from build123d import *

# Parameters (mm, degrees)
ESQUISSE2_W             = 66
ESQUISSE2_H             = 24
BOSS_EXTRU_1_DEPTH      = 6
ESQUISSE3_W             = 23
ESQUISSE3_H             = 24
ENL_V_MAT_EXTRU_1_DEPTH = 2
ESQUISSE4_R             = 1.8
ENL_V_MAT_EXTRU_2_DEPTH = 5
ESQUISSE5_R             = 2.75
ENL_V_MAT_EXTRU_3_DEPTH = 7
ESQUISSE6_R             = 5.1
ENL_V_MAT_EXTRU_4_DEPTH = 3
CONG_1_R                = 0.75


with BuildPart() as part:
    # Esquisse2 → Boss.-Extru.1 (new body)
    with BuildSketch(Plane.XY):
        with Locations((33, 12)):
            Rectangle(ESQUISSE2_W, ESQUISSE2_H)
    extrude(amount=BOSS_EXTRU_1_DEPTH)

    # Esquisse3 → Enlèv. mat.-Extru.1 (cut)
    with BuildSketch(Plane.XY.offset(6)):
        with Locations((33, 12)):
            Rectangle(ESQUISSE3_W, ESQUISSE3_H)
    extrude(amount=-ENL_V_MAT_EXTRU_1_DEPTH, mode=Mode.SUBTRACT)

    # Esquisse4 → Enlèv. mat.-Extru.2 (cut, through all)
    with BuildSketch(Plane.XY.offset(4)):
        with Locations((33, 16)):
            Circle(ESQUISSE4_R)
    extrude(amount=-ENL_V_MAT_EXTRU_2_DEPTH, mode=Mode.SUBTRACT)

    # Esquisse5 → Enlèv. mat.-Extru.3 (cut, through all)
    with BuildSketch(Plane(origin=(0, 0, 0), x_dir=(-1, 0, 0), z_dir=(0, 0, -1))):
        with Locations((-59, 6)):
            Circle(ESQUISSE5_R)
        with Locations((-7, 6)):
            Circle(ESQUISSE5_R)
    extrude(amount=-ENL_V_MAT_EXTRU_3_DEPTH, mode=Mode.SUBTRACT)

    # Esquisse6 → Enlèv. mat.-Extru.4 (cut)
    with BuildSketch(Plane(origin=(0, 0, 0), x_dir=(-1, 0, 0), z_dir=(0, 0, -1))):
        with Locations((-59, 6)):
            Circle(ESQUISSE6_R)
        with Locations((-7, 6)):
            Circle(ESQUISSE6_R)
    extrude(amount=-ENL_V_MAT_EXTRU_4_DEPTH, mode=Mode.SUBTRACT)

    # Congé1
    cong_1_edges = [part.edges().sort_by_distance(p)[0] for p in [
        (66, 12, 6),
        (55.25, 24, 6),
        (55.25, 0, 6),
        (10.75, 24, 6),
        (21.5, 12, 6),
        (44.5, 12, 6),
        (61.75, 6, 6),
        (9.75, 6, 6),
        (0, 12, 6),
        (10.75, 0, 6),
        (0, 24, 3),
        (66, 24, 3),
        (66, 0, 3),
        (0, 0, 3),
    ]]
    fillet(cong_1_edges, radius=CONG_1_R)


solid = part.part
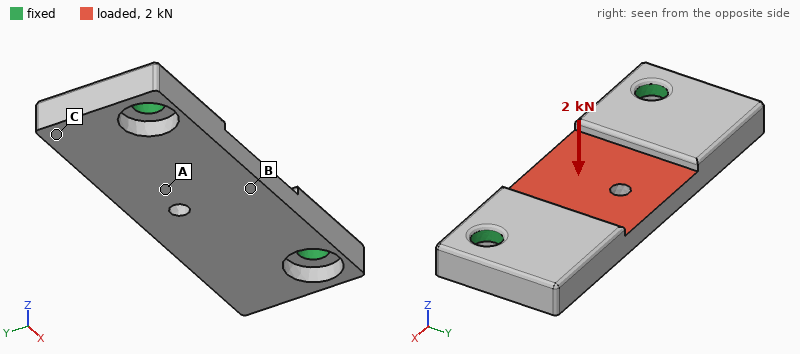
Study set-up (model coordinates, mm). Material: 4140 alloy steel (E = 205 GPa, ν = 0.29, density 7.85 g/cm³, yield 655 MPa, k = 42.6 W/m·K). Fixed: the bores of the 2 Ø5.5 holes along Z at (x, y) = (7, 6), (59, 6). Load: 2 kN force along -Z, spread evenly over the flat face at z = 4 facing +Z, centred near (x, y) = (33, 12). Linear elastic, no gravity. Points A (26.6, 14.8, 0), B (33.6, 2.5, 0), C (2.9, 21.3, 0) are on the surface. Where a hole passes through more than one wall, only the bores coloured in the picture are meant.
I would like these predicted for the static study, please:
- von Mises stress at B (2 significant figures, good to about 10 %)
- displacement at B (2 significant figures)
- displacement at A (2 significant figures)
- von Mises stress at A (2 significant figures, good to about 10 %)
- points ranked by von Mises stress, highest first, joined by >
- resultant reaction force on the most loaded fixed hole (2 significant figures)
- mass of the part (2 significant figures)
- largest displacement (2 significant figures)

140 MPa
36 µm
50 µm
80 MPa
B > A > C
2.3 kN
60 g
72 µm
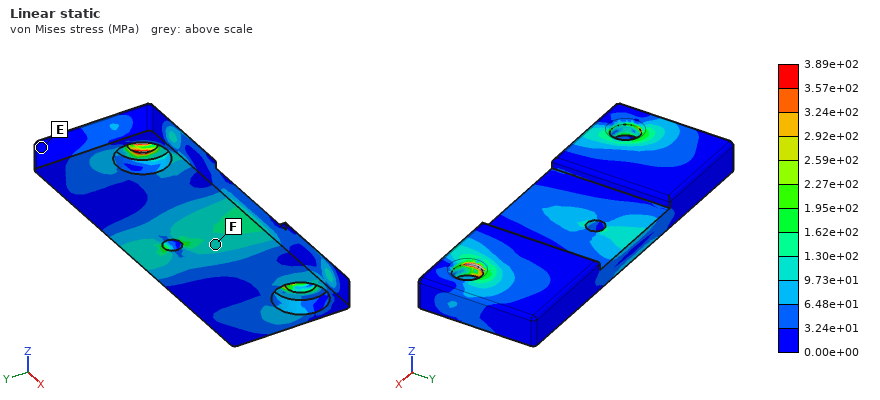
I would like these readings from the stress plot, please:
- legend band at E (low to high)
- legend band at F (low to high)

0.00e+00 to 3.24e+01 MPa
9.73e+01 to 1.30e+02 MPa
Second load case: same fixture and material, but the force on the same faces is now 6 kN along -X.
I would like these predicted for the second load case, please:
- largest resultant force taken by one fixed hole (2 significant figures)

3.1 kN
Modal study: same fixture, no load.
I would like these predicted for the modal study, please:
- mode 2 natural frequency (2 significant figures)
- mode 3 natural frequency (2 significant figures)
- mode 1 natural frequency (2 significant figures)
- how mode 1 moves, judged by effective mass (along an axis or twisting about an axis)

9600 Hz
9900 Hz
5700 Hz
along Z
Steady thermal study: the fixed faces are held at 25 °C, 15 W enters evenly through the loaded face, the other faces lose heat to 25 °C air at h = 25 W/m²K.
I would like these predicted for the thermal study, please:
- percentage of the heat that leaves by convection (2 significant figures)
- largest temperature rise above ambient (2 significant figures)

11 %
37 K
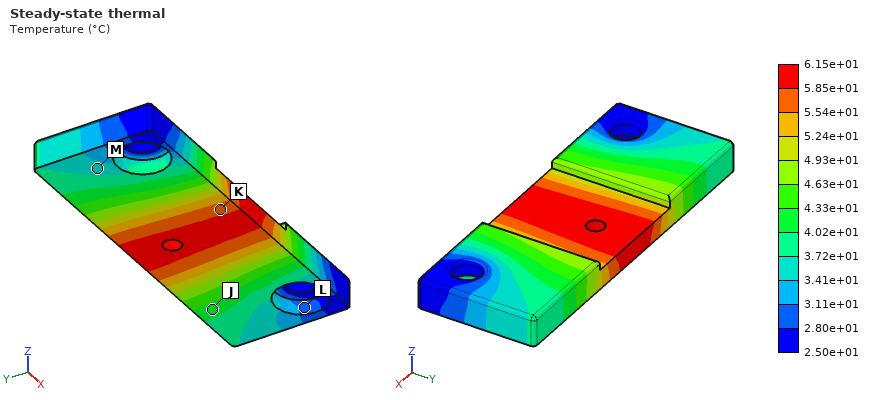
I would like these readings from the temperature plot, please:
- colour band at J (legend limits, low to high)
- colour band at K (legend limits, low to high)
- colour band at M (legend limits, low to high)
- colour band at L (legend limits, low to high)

4.02e+01 to 4.33e+01 °C
5.54e+01 to 5.85e+01 °C
3.41e+01 to 3.72e+01 °C
2.80e+01 to 3.11e+01 °C
